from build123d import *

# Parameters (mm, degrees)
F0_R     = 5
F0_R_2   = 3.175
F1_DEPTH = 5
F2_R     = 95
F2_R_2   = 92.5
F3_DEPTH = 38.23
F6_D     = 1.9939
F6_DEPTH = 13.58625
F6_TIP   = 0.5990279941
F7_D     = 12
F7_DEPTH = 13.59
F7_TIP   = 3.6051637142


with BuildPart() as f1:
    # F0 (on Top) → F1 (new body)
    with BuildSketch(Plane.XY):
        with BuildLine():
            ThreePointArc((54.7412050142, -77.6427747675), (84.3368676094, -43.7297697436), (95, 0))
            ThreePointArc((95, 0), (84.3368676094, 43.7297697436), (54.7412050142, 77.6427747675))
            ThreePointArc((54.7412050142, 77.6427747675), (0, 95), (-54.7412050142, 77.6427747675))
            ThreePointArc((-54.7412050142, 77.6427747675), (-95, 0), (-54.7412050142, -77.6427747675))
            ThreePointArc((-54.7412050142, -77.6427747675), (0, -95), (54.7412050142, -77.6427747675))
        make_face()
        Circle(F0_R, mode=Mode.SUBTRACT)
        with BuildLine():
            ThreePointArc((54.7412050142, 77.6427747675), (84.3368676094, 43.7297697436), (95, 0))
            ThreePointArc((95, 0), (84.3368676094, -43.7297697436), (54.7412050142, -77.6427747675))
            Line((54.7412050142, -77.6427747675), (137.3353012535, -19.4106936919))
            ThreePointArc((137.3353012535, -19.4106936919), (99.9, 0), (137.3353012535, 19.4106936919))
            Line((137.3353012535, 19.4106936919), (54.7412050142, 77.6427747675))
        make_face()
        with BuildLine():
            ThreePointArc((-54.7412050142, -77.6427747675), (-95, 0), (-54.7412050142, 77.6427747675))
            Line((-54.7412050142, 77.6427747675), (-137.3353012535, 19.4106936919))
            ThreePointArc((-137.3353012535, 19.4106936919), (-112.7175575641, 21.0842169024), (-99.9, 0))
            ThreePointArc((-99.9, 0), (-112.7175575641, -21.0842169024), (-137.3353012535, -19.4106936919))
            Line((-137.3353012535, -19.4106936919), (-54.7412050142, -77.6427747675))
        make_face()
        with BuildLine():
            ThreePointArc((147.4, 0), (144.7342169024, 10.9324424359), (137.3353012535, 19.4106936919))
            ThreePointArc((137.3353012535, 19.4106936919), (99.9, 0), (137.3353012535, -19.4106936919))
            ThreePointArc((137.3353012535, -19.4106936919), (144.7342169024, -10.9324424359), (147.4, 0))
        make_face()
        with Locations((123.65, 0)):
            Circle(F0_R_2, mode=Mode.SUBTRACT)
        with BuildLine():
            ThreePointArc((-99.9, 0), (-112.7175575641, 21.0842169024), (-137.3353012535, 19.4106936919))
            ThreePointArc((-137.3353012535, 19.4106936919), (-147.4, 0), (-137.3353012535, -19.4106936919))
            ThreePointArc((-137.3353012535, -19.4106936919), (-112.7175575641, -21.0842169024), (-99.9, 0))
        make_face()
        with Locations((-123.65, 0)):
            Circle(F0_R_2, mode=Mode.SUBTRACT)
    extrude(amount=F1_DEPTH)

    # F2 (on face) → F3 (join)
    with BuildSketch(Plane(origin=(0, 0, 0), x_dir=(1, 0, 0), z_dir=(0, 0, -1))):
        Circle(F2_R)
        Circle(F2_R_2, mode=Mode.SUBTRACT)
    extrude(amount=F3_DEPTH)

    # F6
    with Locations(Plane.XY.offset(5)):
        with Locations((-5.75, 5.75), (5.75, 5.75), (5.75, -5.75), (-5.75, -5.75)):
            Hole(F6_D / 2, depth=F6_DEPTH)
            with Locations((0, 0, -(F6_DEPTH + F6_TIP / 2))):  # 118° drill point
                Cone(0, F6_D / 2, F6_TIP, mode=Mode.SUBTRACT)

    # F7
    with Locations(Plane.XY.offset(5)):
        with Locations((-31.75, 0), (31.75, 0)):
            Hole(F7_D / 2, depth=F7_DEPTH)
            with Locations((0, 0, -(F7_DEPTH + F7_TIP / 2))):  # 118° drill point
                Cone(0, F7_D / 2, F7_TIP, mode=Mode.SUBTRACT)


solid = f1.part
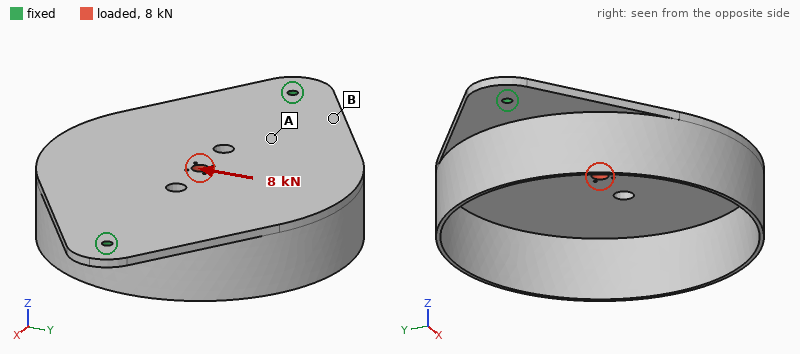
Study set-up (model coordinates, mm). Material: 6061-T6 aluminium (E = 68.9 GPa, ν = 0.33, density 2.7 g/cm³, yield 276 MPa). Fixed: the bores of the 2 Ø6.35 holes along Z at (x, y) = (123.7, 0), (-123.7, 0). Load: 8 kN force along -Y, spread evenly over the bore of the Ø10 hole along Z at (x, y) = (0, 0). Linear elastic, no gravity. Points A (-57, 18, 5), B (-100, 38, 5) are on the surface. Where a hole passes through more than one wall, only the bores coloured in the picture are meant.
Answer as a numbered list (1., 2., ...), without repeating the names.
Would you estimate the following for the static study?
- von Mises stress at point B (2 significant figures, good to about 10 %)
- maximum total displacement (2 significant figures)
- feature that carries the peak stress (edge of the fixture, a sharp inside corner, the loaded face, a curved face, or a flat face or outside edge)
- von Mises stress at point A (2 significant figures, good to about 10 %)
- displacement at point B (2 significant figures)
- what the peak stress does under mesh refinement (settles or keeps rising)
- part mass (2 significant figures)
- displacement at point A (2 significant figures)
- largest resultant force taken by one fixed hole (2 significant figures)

1. 17 MPa
2. 65 µm
3. edge of the fixture
4. 6.4 MPa
5. 24 µm
6. keeps rising
7. 640 g
8. 40 µm
9. 4.0 kN
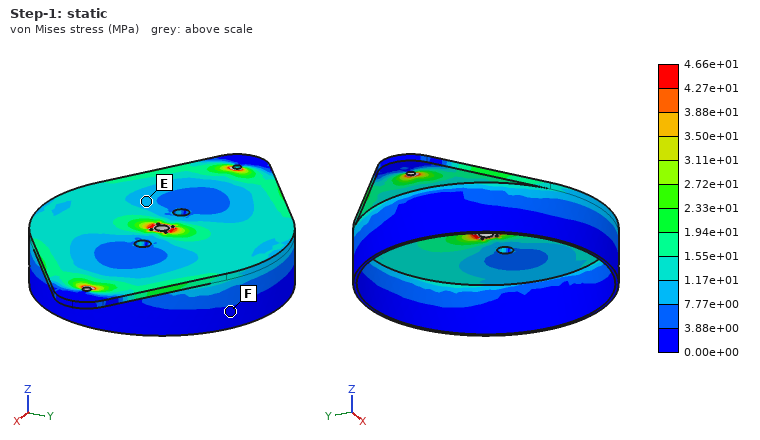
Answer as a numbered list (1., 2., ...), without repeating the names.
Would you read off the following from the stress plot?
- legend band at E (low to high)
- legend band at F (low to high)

1. 7.77e+00 to 1.17e+01 MPa
2. 0.00e+00 to 3.88e+00 MPa
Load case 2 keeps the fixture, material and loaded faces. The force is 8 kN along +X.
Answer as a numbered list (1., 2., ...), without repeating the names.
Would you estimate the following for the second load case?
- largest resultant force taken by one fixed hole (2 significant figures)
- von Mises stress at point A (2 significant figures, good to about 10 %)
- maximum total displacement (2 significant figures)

1. 4.0 kN
2. 12 MPa
3. 35 µm
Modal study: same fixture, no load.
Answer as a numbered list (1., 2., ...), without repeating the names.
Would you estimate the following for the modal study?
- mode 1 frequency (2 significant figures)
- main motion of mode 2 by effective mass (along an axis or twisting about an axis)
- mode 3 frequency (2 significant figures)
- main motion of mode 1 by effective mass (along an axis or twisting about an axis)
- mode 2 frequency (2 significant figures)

1. 240 Hz
2. along Z
3. 860 Hz
4. twisting about X
5. 330 Hz
